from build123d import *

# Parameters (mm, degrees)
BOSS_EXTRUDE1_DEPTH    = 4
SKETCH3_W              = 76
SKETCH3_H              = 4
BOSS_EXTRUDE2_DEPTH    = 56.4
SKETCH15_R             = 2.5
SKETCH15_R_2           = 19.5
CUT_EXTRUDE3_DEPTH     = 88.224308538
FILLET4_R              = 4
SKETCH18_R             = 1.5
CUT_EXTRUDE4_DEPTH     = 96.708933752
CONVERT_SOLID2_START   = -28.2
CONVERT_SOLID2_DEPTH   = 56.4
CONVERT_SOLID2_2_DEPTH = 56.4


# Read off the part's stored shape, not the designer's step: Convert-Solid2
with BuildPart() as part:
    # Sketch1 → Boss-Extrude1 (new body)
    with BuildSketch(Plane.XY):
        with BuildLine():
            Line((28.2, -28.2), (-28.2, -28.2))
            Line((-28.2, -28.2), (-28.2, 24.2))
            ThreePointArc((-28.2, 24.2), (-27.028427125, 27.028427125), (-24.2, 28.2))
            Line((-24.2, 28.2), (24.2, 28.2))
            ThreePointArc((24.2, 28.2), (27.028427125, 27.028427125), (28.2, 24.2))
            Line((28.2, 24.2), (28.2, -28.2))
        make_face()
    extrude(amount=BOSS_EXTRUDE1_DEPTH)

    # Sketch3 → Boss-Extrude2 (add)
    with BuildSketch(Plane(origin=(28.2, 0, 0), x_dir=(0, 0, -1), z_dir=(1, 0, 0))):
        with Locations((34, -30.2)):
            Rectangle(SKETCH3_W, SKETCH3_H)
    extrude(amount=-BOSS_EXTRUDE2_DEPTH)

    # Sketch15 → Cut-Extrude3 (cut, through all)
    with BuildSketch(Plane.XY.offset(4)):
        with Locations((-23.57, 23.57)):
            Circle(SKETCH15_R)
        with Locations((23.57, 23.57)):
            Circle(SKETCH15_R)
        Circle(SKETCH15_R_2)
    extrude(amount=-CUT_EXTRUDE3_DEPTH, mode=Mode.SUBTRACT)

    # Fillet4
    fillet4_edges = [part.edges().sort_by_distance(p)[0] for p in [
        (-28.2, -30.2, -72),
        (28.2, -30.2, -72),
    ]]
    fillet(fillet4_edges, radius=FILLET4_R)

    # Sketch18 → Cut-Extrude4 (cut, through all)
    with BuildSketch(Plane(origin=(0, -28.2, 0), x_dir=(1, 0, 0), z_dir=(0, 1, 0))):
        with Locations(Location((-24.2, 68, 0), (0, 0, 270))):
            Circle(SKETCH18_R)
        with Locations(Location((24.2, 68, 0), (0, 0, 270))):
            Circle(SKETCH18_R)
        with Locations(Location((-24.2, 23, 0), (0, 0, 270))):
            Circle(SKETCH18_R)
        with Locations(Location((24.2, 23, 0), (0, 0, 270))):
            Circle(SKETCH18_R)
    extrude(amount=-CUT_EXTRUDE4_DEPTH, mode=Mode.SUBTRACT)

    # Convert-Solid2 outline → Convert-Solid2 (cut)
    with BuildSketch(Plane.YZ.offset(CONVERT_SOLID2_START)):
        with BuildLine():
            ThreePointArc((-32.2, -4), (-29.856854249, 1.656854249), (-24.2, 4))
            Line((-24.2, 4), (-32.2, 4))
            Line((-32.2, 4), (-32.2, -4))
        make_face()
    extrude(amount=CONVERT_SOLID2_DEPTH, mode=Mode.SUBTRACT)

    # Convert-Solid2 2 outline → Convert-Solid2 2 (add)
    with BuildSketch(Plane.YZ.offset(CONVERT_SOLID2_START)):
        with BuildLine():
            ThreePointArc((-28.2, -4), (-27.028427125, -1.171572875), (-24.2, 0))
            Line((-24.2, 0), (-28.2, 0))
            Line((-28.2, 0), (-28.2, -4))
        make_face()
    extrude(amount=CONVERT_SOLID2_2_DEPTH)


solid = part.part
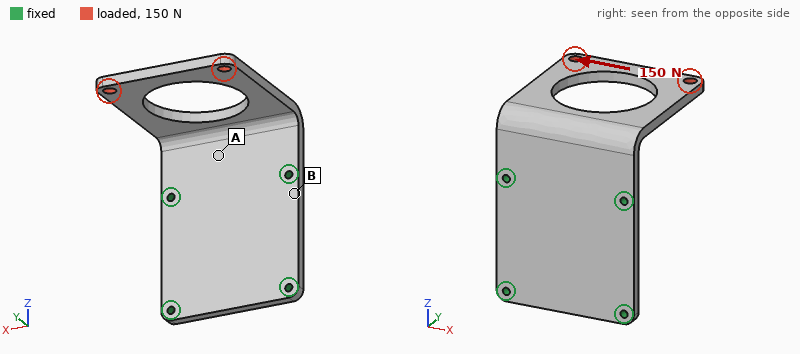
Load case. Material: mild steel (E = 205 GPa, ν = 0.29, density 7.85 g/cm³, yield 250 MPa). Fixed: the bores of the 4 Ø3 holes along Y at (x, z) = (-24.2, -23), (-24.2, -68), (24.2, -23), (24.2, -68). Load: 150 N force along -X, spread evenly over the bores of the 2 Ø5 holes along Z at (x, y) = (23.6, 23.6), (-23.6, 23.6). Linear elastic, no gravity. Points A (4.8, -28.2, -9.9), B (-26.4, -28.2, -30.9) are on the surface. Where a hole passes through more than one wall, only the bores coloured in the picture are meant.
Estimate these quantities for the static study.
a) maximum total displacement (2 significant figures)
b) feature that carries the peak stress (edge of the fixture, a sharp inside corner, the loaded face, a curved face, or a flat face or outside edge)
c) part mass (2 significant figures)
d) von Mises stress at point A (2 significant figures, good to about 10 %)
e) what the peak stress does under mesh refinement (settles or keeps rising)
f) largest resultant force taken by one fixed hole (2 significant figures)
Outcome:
63 µm
edge of the fixture
190 g
21 MPa
keeps rising
210 N
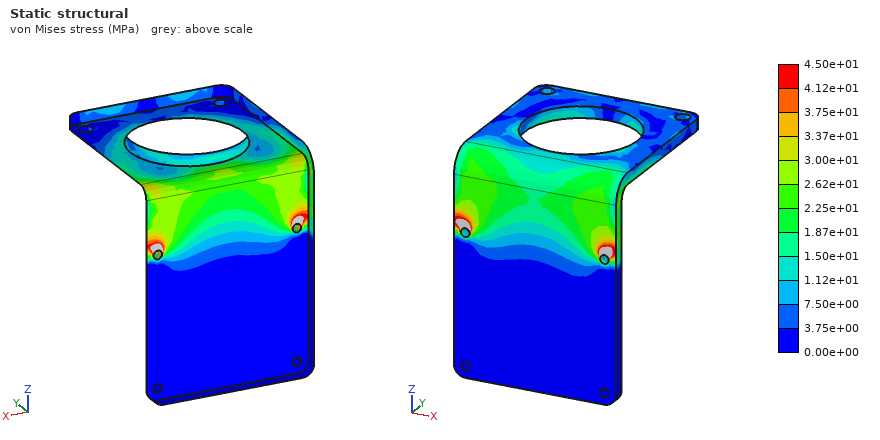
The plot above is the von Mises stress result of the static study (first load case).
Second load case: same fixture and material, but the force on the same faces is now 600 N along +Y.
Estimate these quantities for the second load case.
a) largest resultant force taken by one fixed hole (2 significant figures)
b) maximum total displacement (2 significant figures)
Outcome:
360 N
0.24 mm
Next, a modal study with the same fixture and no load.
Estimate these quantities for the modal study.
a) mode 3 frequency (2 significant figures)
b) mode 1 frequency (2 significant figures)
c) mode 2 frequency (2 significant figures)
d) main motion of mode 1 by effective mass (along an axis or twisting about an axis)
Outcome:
2100 Hz
610 Hz
1400 Hz
along Z
